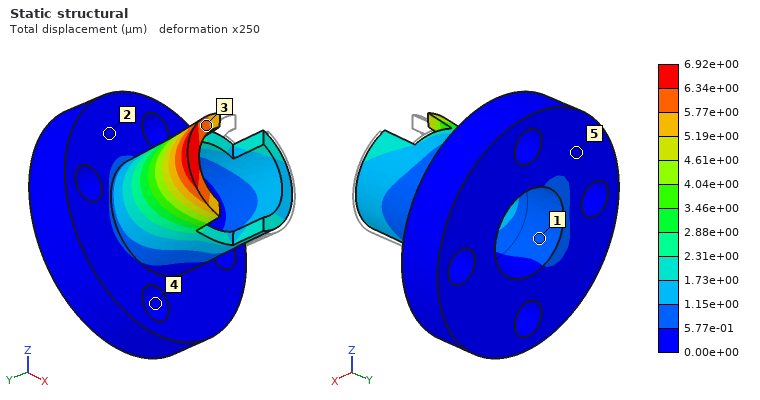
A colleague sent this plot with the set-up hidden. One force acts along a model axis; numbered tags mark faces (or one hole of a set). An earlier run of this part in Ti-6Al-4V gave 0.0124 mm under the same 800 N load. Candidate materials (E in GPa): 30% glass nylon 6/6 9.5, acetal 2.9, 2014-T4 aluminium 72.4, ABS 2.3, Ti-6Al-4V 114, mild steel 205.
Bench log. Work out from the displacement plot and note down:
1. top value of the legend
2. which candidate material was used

6.92e+00 µm
mild steel
